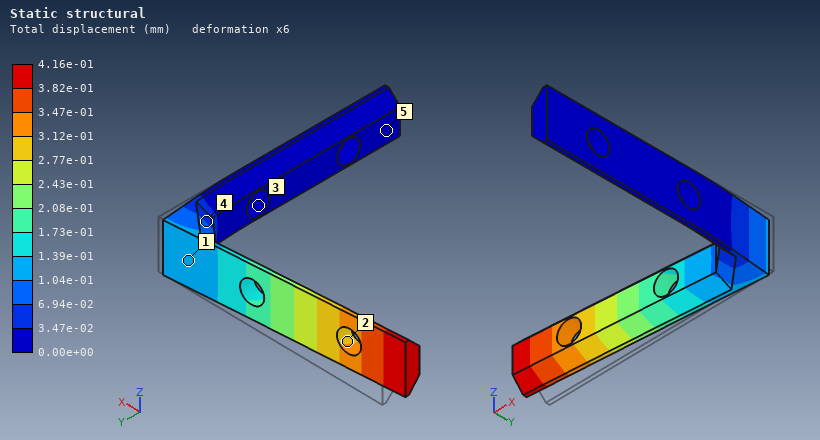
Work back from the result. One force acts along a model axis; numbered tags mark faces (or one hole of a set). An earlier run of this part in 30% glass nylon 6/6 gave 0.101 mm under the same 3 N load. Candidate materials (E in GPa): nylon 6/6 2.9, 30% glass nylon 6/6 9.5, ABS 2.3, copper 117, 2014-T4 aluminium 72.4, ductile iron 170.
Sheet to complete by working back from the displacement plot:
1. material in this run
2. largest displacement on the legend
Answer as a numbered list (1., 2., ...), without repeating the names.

1. ABS
2. 4.16e-01 mm
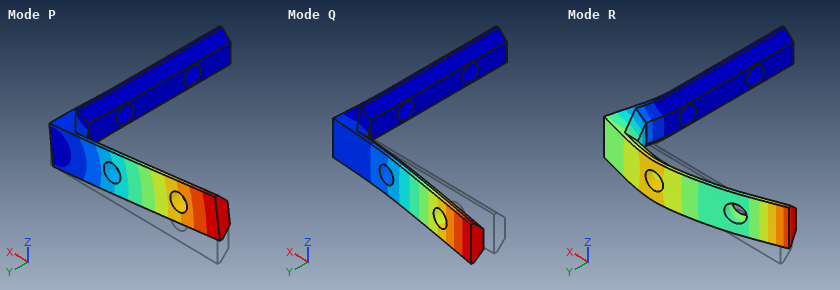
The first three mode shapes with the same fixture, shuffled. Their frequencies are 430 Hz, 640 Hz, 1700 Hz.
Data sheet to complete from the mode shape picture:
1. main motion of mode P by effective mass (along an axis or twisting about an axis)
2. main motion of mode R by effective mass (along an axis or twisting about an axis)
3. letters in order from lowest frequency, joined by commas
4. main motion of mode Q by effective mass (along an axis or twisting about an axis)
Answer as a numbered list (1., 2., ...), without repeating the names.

1. along Z
2. along X
3. Q, P, R
4. along Y
